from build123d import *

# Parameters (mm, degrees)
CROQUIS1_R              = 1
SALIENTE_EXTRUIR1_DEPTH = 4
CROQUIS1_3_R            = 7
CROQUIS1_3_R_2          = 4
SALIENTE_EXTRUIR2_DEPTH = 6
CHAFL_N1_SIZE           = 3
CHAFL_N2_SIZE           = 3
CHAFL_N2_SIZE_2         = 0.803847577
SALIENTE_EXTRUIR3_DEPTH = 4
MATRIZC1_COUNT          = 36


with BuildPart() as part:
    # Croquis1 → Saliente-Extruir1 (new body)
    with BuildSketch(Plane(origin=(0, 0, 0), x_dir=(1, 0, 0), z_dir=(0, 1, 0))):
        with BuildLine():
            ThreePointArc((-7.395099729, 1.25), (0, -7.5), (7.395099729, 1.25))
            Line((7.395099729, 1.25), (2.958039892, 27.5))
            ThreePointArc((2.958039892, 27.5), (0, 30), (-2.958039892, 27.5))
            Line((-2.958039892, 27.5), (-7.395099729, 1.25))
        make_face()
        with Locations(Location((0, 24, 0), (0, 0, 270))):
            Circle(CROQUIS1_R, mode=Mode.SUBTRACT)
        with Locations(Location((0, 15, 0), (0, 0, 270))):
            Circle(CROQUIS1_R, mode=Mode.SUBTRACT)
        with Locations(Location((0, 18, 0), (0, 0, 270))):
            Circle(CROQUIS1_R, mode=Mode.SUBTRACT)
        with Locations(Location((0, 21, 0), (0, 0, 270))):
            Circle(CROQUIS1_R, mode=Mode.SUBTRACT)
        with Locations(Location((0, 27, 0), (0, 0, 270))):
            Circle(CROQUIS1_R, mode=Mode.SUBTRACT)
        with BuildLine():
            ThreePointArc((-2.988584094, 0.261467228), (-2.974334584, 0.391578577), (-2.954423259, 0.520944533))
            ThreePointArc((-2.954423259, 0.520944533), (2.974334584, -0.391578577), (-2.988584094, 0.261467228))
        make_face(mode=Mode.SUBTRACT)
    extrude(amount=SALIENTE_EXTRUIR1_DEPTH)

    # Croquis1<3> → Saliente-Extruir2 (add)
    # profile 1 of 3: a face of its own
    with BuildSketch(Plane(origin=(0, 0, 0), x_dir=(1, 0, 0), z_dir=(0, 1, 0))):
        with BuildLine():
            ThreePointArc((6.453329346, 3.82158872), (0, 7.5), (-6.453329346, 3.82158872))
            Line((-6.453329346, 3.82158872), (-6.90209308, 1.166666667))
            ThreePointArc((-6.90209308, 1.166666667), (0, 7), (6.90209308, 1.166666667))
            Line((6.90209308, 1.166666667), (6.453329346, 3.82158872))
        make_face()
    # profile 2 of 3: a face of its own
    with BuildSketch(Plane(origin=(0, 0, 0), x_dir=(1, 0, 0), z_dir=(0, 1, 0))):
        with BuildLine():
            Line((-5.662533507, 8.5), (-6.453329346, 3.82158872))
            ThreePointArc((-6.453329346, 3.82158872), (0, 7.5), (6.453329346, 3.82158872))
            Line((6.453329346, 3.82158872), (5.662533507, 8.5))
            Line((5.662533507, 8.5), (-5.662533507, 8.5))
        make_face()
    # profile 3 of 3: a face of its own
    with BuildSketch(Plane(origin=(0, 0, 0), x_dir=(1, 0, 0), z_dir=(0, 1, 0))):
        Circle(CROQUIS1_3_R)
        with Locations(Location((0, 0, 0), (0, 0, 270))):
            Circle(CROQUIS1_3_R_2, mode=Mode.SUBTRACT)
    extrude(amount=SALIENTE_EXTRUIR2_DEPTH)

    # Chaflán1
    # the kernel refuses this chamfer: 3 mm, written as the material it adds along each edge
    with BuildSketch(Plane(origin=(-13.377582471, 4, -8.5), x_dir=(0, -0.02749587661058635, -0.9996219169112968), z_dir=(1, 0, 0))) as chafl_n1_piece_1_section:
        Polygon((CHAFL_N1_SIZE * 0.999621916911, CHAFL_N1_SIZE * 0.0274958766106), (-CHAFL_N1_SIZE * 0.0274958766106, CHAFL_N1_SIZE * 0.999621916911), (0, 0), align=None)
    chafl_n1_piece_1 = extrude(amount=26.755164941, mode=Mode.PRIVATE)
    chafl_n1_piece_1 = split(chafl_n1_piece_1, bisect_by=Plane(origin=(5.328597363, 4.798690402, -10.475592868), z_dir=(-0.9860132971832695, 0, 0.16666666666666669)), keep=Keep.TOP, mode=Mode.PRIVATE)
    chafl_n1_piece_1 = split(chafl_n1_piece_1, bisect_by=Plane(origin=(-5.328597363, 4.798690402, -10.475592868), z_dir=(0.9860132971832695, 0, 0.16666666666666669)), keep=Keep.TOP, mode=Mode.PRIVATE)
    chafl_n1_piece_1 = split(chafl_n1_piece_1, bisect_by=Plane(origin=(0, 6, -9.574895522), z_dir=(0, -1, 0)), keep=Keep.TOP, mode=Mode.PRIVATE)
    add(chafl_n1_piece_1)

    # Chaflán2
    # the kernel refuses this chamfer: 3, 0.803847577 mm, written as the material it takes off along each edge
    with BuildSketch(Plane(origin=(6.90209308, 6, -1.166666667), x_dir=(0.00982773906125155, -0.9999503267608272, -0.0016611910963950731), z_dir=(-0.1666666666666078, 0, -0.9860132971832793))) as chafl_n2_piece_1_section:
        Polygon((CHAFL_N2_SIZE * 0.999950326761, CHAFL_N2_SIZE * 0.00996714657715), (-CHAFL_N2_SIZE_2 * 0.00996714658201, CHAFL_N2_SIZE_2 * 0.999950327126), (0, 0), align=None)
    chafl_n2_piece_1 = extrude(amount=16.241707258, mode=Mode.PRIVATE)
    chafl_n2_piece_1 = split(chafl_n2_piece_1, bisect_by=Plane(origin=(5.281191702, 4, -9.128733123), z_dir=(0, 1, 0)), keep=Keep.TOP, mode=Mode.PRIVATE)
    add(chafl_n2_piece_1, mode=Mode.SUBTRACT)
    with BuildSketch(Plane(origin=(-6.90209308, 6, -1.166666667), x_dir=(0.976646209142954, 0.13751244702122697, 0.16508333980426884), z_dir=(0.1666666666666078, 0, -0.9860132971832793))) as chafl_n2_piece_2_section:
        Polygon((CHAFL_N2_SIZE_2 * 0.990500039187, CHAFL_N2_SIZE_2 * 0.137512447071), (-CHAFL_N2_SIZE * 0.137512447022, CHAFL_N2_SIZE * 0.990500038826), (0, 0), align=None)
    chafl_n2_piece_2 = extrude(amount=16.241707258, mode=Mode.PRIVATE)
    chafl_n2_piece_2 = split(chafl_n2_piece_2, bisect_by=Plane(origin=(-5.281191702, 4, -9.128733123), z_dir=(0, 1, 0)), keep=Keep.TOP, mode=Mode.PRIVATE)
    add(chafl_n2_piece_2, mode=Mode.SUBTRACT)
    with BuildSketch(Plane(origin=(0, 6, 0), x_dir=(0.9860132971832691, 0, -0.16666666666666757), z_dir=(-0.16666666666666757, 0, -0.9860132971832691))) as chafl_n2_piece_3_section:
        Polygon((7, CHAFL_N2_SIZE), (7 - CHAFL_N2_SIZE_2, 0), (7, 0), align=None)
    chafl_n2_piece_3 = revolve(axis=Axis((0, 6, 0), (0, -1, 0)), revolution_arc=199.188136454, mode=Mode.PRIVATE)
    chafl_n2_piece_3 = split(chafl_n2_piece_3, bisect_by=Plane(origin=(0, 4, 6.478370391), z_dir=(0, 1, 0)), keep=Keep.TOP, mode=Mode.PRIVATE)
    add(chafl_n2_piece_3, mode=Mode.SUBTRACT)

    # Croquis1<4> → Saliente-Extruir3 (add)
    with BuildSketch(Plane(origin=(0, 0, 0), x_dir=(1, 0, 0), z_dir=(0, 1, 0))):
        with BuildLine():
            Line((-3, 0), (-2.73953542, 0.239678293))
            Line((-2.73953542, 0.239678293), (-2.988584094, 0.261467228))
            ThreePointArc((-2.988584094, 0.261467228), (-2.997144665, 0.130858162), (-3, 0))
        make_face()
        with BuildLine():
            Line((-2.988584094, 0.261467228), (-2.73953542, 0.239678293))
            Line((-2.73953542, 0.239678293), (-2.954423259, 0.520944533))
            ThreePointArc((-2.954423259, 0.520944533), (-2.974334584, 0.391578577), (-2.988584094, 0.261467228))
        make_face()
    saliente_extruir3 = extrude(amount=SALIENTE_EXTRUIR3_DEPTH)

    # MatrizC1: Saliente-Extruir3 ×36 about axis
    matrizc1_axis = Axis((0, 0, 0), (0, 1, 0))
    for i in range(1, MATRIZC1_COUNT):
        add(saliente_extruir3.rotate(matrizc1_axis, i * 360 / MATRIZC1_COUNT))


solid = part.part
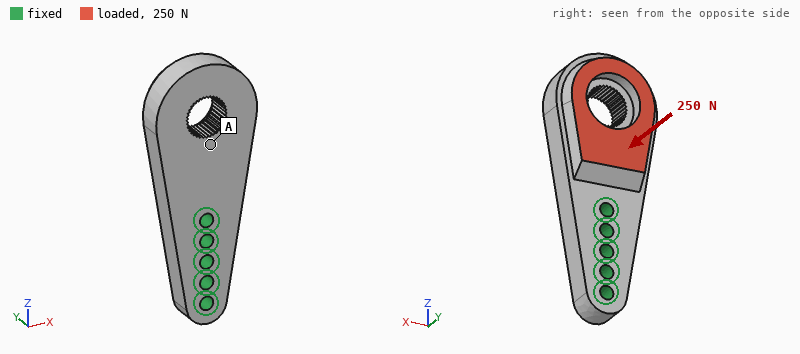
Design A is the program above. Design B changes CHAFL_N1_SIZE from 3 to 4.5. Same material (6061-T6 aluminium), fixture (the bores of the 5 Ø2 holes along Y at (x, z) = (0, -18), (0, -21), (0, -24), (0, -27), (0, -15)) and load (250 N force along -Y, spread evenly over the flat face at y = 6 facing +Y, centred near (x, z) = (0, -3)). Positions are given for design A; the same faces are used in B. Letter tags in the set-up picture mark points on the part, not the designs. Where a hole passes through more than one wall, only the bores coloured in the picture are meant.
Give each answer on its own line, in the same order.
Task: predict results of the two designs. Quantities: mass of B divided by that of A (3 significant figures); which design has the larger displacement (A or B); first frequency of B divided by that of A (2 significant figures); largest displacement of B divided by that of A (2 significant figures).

1.02
A
1.1
0.83
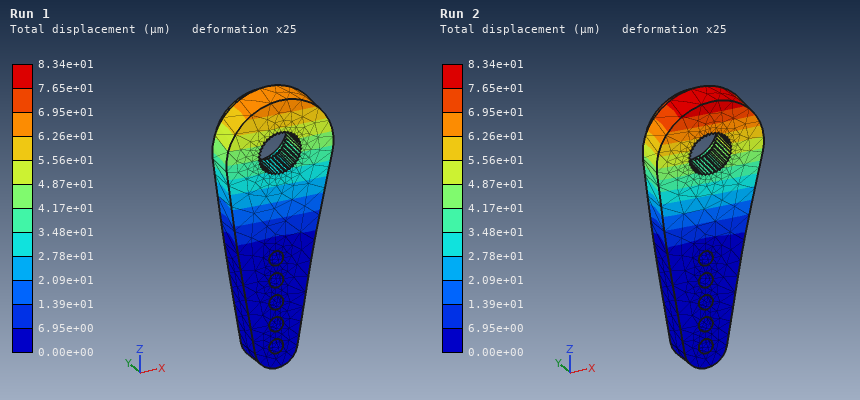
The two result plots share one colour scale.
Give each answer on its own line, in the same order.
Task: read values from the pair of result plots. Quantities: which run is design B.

Run 1
